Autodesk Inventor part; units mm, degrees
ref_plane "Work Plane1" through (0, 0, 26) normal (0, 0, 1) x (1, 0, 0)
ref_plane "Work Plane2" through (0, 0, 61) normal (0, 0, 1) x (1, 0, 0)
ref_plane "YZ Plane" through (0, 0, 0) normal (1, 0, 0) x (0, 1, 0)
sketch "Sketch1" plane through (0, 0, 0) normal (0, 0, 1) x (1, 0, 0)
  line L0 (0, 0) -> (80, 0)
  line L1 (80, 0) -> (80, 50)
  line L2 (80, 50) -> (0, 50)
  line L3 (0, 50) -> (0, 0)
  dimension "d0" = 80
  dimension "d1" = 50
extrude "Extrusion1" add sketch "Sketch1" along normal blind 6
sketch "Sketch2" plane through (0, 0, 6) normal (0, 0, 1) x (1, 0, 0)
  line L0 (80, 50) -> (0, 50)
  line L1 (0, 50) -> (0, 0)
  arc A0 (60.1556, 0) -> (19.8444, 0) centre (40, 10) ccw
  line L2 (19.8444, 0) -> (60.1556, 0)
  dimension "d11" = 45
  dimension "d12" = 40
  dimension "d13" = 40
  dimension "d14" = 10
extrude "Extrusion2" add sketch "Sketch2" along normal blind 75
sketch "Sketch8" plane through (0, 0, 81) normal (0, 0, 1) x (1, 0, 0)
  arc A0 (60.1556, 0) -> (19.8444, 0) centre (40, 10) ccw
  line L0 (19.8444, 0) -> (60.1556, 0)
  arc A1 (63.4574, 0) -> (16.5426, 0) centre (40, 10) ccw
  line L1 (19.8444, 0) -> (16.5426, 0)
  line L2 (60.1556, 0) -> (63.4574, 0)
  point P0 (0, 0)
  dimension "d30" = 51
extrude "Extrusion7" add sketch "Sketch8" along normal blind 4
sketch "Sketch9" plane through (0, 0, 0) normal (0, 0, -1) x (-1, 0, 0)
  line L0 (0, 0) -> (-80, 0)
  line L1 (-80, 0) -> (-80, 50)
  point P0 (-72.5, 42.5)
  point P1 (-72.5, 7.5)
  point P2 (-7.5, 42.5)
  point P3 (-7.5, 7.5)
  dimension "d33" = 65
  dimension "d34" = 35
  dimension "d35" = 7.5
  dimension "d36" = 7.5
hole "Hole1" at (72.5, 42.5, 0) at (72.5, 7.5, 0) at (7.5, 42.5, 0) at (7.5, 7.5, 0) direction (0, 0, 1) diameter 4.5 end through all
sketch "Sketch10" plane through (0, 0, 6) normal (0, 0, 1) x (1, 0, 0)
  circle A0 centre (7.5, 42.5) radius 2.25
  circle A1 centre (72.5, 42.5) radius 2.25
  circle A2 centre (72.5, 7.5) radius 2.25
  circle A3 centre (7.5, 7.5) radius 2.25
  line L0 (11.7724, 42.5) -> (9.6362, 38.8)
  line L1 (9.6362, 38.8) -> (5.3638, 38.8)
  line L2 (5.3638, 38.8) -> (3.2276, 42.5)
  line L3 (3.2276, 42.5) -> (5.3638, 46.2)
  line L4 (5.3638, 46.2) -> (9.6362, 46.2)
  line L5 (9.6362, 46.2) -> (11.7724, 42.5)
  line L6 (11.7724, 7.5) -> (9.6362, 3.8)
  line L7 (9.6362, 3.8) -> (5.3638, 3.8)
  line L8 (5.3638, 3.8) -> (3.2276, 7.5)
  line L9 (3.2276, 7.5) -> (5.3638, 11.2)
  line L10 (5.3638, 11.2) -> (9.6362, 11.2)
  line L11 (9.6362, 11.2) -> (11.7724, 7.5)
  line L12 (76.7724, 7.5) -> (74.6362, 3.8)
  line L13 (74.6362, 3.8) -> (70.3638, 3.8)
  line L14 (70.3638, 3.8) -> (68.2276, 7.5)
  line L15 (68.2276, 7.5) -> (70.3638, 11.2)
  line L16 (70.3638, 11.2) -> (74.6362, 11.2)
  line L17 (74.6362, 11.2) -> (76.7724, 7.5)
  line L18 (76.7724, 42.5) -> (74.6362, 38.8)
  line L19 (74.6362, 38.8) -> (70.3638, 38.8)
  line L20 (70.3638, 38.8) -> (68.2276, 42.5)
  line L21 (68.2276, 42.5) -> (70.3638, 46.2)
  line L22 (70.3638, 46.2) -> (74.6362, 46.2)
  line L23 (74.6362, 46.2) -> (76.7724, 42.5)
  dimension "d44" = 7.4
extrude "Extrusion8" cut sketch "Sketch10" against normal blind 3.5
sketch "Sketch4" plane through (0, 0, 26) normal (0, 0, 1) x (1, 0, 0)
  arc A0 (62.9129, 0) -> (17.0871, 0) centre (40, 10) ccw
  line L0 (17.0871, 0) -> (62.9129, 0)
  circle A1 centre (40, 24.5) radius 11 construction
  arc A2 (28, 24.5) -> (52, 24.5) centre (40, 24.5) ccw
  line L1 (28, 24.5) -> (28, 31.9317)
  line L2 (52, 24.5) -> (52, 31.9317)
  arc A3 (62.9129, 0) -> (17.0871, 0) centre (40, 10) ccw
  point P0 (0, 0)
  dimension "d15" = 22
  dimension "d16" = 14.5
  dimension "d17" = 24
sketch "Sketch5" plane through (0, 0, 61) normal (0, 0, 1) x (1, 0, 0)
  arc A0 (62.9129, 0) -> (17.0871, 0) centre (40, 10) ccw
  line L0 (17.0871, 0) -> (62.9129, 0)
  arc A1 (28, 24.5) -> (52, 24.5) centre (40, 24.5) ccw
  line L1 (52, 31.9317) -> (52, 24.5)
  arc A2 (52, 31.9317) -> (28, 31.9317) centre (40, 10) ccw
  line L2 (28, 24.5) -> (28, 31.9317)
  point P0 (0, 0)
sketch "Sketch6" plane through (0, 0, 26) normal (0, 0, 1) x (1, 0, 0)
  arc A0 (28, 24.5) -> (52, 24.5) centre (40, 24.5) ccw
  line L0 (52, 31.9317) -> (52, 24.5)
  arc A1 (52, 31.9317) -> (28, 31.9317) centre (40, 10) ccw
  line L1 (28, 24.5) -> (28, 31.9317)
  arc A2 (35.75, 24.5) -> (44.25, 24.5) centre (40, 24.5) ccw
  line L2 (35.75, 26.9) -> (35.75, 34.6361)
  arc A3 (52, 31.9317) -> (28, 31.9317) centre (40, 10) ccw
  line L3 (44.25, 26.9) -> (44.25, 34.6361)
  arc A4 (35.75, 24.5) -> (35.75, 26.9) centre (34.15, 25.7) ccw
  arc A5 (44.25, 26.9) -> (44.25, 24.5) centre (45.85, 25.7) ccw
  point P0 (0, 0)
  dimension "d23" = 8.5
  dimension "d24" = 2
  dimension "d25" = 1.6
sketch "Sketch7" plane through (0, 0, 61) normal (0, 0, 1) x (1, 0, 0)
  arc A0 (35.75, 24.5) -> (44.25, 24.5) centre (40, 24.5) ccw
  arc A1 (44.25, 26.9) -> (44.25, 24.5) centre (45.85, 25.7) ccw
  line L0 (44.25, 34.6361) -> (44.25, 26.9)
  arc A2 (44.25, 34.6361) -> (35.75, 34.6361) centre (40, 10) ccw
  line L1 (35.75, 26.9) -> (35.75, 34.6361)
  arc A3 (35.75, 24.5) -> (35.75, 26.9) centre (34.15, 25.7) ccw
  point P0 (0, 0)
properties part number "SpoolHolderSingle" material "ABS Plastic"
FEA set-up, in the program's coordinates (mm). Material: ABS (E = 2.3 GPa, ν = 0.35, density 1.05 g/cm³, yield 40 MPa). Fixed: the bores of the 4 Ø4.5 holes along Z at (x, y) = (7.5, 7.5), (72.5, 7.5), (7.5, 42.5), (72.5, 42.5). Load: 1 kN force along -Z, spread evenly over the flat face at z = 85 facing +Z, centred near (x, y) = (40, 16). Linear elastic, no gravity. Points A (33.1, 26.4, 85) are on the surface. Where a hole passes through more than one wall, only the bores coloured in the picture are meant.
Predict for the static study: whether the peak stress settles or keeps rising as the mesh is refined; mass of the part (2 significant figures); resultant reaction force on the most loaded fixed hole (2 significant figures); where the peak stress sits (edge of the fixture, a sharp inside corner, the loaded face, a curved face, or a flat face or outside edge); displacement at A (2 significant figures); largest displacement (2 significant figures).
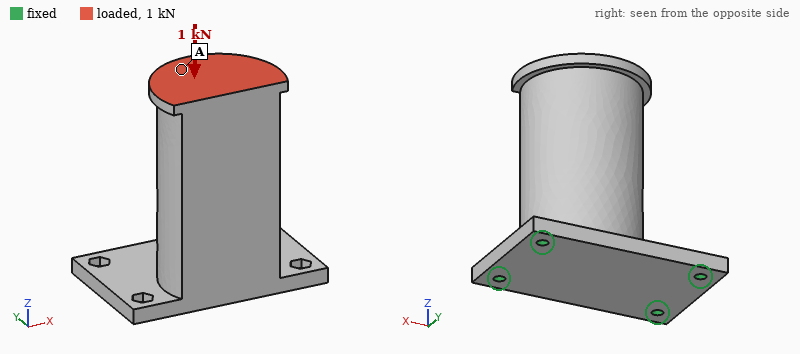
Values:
keeps rising
130 g
540 N
edge of the fixture
0.35 mm
0.37 mm
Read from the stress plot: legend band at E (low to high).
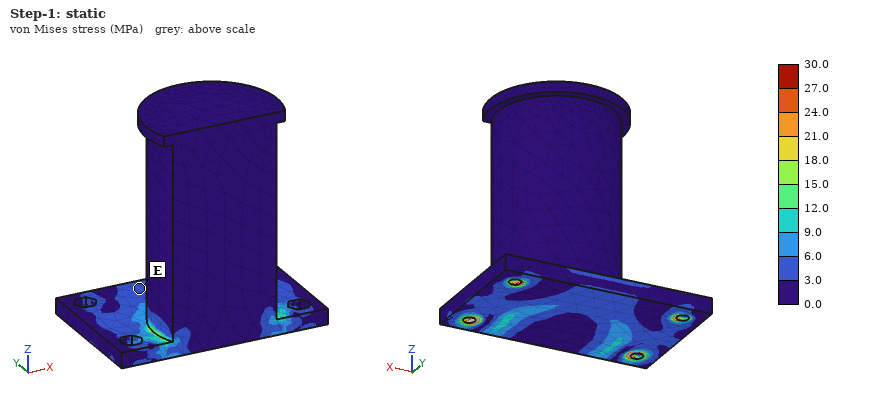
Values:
3.0 to 6.0 MPa
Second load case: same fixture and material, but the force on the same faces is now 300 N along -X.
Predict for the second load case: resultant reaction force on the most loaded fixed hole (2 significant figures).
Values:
390 N
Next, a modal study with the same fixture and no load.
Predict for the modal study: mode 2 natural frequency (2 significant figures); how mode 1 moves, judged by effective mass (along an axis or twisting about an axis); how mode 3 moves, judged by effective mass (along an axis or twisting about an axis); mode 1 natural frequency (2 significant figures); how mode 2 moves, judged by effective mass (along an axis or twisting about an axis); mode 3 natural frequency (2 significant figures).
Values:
520 Hz
along Y
along Z
260 Hz
along X
930 Hz
